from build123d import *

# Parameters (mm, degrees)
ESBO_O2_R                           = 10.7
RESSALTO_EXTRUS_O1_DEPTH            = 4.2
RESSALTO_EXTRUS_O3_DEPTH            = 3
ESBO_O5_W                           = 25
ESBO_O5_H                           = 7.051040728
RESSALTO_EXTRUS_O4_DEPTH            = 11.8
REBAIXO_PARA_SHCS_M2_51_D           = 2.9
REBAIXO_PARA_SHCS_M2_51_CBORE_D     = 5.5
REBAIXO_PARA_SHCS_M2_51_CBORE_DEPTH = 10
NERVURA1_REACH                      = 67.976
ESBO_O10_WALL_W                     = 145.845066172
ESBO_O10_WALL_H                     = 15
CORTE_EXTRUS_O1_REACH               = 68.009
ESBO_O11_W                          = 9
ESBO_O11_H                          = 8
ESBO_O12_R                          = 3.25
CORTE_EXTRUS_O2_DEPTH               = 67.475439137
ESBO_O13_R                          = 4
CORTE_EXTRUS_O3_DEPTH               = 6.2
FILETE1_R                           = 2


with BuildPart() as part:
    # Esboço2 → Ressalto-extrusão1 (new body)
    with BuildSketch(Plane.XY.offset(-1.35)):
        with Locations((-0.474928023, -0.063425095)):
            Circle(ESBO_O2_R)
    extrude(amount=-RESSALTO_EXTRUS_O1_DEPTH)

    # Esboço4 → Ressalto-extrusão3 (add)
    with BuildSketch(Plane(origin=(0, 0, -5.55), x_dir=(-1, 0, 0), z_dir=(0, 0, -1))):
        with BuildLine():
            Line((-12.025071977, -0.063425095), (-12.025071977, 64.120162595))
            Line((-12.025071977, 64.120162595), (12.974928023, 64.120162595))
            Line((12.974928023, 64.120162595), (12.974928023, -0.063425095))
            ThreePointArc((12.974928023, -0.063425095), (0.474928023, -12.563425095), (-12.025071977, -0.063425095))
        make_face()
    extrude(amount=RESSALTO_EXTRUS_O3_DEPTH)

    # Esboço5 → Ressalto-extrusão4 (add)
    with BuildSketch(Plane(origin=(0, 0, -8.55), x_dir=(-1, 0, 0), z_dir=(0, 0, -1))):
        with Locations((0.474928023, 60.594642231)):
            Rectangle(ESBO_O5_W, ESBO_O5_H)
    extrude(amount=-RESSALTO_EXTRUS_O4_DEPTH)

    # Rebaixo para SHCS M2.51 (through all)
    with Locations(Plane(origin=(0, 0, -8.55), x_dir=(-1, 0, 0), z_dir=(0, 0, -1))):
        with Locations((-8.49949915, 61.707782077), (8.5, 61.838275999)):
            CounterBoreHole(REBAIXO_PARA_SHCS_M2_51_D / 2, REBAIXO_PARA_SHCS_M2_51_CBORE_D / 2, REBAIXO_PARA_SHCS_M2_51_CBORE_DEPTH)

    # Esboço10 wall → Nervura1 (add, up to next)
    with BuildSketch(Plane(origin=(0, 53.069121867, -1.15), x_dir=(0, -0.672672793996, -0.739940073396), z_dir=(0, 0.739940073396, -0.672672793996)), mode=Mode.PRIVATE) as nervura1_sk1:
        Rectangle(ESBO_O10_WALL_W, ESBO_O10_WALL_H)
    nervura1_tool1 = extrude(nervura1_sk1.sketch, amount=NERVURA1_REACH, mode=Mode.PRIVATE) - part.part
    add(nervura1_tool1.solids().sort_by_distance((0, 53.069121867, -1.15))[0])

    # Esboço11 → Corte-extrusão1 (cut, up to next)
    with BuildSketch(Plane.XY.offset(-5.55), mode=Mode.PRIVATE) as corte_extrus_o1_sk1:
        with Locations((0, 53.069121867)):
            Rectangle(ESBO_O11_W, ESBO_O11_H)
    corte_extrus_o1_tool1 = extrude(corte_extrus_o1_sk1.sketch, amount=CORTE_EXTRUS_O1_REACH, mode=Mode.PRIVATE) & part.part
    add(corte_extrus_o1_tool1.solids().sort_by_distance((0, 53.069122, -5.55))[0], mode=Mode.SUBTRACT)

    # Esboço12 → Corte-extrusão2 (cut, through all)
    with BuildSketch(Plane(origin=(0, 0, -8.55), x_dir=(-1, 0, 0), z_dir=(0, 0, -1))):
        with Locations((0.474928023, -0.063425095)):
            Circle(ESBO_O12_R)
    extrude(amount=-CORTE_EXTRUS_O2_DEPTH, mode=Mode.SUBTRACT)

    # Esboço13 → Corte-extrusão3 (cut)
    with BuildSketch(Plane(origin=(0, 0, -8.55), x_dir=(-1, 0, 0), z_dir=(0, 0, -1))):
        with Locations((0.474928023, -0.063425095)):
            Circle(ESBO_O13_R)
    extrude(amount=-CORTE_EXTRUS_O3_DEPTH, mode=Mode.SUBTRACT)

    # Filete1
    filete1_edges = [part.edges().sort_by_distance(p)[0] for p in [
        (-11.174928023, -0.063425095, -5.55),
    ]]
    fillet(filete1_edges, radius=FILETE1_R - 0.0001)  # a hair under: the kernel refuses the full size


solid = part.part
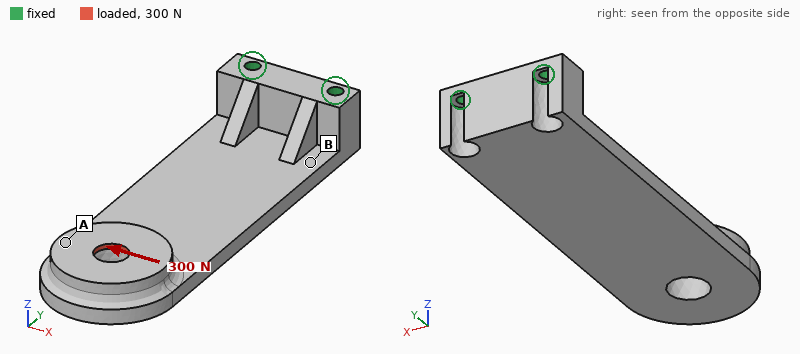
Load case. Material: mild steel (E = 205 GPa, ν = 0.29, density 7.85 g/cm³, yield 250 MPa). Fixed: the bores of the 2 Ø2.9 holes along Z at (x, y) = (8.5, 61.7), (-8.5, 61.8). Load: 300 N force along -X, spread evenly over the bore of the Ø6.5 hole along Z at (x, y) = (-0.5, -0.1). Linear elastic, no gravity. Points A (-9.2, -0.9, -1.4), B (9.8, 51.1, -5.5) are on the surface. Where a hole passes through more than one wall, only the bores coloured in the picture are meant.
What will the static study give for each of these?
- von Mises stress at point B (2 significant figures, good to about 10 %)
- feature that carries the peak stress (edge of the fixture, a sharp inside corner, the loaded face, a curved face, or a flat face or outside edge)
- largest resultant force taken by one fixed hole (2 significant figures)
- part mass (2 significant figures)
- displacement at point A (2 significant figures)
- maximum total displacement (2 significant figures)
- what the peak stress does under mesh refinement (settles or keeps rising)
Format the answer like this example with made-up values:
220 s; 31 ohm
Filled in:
50 MPa; edge of the fixture; 1.0 kN; 63 g; 0.15 mm; 0.16 mm; keeps rising
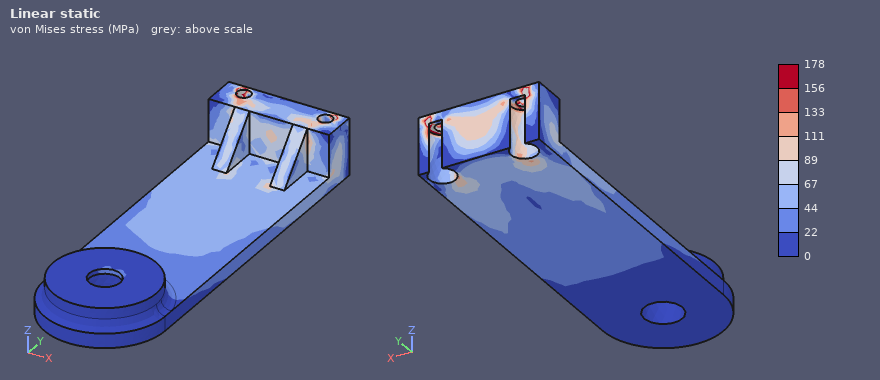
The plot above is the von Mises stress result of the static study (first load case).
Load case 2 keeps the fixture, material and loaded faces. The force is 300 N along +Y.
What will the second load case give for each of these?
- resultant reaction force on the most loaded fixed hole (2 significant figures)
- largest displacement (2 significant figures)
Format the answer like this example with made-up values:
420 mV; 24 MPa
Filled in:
160 N; 0.21 mm
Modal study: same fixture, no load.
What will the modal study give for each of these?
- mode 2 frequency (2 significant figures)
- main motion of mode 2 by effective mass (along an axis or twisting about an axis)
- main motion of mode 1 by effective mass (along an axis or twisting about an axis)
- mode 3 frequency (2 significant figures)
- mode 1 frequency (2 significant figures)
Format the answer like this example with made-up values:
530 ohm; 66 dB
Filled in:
1600 Hz; along X; along Z; 2500 Hz; 420 Hz
